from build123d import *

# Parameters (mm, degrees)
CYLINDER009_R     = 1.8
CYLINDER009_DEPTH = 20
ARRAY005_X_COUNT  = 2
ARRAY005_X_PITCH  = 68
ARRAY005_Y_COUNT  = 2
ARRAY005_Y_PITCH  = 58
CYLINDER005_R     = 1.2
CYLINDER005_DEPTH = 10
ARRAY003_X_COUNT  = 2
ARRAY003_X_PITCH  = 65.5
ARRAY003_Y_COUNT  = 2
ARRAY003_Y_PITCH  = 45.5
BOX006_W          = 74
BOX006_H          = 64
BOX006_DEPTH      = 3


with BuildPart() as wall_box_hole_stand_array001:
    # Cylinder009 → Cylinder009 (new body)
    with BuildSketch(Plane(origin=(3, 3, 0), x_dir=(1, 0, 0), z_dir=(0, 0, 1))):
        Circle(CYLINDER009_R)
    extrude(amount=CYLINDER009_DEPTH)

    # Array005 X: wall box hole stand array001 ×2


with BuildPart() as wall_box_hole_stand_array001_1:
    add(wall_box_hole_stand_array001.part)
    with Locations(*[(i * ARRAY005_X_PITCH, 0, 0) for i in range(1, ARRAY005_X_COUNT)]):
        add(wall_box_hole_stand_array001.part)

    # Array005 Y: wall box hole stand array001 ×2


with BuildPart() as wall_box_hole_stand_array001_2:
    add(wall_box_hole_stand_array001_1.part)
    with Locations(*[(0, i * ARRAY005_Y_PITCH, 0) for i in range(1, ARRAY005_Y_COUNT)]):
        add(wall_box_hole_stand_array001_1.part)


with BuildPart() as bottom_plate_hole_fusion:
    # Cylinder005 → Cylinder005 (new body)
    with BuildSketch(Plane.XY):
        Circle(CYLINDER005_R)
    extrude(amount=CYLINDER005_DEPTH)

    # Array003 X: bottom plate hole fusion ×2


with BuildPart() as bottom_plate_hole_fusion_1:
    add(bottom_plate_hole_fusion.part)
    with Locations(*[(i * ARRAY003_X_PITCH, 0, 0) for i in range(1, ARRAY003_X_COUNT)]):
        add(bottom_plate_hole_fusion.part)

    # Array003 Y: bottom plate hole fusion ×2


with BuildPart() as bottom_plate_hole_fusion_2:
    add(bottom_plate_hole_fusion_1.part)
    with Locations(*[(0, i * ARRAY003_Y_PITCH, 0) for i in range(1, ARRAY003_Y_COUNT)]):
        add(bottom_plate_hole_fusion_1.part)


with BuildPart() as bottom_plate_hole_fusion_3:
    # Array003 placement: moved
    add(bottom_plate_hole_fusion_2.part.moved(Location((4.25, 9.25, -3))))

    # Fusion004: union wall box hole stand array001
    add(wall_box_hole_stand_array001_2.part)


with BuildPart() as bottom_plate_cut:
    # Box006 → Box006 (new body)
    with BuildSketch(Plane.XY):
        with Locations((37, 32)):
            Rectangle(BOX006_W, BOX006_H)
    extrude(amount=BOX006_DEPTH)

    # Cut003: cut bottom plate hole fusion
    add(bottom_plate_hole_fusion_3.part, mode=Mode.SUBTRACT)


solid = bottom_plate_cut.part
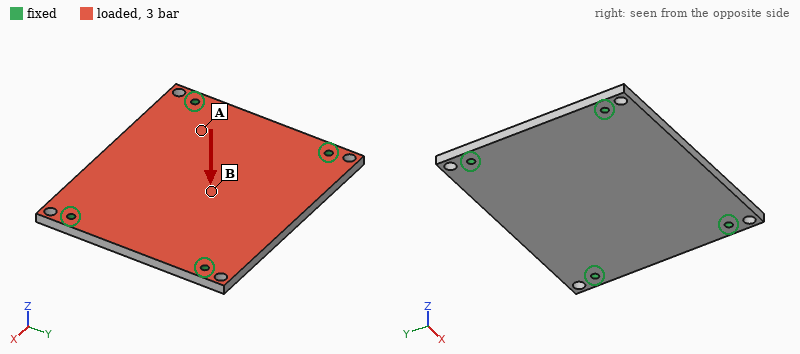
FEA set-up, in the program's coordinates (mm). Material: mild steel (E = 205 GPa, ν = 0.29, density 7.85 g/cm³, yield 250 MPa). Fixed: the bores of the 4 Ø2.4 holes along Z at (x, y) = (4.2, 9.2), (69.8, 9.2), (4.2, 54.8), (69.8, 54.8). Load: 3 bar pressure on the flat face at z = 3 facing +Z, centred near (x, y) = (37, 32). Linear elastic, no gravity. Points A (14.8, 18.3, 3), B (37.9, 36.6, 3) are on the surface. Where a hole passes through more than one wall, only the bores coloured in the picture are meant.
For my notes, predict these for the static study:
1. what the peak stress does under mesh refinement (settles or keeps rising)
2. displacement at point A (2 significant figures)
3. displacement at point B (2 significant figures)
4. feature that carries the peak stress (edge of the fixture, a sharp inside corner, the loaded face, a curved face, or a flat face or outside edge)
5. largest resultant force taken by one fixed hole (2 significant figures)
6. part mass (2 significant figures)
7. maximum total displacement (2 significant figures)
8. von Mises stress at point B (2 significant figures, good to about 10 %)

keeps rising
24 µm
54 µm
edge of the fixture
350 N
110 g
55 µm
39 MPa
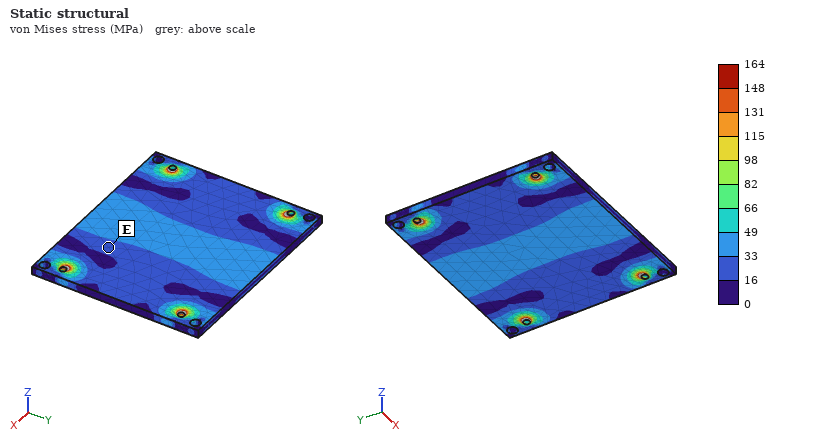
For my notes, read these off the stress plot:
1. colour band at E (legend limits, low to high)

16 to 33 MPa
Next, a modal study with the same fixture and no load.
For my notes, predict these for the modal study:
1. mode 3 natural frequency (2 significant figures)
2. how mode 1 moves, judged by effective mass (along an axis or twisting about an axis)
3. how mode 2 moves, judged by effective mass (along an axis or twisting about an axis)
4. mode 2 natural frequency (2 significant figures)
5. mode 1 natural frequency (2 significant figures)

5700 Hz
along Z
twisting about X
4000 Hz
2900 Hz
